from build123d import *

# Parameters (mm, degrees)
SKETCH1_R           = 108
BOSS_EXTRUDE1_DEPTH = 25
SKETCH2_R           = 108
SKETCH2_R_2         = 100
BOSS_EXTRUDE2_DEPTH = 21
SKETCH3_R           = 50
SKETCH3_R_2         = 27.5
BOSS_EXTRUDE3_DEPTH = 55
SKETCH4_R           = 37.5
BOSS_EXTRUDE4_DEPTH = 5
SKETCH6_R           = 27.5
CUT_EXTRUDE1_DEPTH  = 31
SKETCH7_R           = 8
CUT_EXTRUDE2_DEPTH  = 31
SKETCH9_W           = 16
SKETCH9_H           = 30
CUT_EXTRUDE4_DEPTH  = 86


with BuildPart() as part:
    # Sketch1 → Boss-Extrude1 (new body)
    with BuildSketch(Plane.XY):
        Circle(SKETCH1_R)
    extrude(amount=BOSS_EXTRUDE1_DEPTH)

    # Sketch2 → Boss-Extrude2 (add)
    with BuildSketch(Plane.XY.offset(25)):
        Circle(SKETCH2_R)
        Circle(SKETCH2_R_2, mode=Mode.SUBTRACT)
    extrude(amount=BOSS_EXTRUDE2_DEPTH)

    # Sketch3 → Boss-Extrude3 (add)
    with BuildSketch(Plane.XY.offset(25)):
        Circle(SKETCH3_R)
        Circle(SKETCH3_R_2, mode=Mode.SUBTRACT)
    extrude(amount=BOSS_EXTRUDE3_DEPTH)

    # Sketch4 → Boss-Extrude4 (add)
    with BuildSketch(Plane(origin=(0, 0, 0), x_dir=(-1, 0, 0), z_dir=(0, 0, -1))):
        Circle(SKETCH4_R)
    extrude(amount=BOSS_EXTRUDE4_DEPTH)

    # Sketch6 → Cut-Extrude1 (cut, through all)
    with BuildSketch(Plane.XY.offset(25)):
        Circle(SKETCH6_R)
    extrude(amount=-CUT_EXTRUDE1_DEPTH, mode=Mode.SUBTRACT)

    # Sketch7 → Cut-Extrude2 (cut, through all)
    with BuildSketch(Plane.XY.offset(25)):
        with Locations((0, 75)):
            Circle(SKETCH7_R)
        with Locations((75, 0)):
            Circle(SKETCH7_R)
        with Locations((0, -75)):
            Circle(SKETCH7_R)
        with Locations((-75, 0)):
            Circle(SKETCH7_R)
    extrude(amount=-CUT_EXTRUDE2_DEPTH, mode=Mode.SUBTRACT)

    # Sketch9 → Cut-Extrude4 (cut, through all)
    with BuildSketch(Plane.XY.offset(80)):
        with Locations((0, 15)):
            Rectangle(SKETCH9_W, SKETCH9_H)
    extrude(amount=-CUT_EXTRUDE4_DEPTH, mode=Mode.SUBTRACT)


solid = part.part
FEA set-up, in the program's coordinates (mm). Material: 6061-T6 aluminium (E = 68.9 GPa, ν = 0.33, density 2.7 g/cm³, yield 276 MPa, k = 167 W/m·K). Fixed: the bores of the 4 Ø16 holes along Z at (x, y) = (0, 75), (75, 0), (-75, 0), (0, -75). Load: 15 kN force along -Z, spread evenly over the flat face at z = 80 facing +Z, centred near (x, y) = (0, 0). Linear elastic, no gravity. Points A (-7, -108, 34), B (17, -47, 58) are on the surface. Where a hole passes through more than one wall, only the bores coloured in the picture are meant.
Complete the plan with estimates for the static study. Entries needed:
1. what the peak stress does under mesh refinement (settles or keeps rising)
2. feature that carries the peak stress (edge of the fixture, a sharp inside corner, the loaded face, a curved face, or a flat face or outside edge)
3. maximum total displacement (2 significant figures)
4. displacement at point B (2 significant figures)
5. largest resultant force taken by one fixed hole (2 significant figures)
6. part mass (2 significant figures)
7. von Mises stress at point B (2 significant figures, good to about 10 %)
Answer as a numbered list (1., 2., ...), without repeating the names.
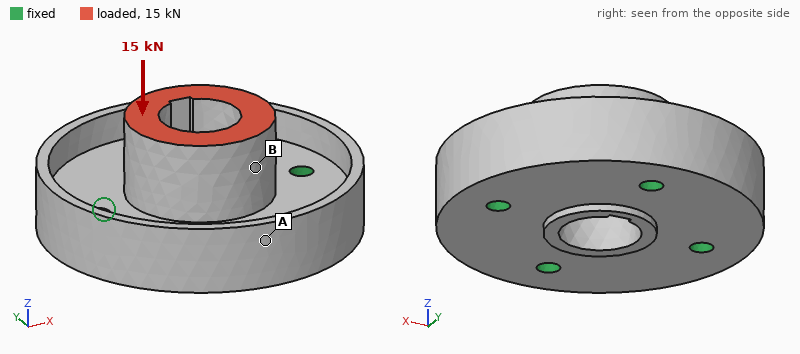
1. keeps rising
2. edge of the fixture
3. 8.3 µm
4. 7.4 µm
5. 3.9 kN
6. 3.4 kg
7. 2.6 MPa
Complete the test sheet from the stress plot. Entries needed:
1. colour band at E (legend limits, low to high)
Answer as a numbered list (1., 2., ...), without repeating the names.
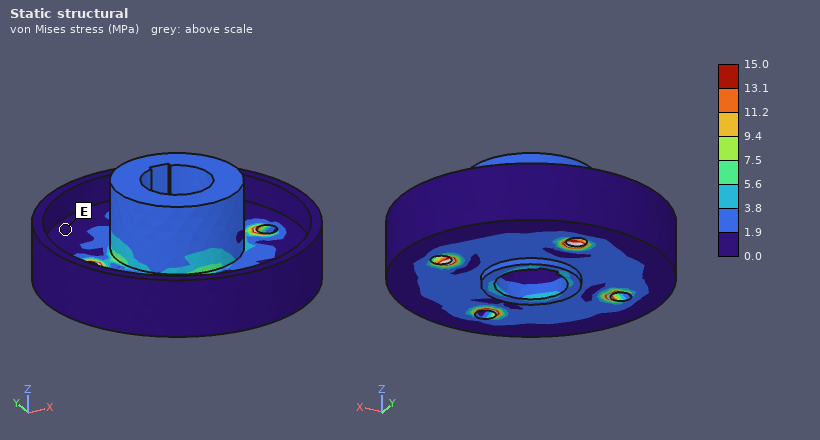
1. 0.0 to 1.9 MPa
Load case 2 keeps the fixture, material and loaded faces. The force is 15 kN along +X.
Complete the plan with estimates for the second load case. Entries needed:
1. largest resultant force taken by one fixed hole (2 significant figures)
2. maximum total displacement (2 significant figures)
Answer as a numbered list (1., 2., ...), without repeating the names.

1. 8.6 kN
2. 33 µm
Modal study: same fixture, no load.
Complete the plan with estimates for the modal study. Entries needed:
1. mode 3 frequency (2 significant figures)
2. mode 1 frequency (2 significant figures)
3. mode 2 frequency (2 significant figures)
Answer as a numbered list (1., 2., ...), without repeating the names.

1. 5200 Hz
2. 4800 Hz
3. 5200 Hz
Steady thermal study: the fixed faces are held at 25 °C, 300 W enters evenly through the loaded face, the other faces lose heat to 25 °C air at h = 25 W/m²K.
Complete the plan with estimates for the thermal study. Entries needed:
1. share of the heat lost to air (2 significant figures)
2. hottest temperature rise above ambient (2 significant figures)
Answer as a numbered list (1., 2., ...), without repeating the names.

1. 7.3 %
2. 28 K
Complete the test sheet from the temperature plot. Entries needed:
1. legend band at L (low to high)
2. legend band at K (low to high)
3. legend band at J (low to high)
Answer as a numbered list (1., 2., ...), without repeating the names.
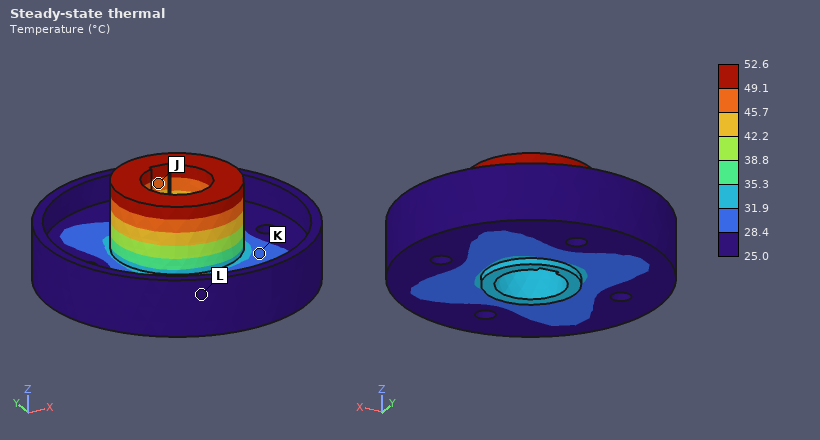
1. 25.0 to 28.4 °C
2. 28.4 to 31.9 °C
3. 45.7 to 49.1 °C
